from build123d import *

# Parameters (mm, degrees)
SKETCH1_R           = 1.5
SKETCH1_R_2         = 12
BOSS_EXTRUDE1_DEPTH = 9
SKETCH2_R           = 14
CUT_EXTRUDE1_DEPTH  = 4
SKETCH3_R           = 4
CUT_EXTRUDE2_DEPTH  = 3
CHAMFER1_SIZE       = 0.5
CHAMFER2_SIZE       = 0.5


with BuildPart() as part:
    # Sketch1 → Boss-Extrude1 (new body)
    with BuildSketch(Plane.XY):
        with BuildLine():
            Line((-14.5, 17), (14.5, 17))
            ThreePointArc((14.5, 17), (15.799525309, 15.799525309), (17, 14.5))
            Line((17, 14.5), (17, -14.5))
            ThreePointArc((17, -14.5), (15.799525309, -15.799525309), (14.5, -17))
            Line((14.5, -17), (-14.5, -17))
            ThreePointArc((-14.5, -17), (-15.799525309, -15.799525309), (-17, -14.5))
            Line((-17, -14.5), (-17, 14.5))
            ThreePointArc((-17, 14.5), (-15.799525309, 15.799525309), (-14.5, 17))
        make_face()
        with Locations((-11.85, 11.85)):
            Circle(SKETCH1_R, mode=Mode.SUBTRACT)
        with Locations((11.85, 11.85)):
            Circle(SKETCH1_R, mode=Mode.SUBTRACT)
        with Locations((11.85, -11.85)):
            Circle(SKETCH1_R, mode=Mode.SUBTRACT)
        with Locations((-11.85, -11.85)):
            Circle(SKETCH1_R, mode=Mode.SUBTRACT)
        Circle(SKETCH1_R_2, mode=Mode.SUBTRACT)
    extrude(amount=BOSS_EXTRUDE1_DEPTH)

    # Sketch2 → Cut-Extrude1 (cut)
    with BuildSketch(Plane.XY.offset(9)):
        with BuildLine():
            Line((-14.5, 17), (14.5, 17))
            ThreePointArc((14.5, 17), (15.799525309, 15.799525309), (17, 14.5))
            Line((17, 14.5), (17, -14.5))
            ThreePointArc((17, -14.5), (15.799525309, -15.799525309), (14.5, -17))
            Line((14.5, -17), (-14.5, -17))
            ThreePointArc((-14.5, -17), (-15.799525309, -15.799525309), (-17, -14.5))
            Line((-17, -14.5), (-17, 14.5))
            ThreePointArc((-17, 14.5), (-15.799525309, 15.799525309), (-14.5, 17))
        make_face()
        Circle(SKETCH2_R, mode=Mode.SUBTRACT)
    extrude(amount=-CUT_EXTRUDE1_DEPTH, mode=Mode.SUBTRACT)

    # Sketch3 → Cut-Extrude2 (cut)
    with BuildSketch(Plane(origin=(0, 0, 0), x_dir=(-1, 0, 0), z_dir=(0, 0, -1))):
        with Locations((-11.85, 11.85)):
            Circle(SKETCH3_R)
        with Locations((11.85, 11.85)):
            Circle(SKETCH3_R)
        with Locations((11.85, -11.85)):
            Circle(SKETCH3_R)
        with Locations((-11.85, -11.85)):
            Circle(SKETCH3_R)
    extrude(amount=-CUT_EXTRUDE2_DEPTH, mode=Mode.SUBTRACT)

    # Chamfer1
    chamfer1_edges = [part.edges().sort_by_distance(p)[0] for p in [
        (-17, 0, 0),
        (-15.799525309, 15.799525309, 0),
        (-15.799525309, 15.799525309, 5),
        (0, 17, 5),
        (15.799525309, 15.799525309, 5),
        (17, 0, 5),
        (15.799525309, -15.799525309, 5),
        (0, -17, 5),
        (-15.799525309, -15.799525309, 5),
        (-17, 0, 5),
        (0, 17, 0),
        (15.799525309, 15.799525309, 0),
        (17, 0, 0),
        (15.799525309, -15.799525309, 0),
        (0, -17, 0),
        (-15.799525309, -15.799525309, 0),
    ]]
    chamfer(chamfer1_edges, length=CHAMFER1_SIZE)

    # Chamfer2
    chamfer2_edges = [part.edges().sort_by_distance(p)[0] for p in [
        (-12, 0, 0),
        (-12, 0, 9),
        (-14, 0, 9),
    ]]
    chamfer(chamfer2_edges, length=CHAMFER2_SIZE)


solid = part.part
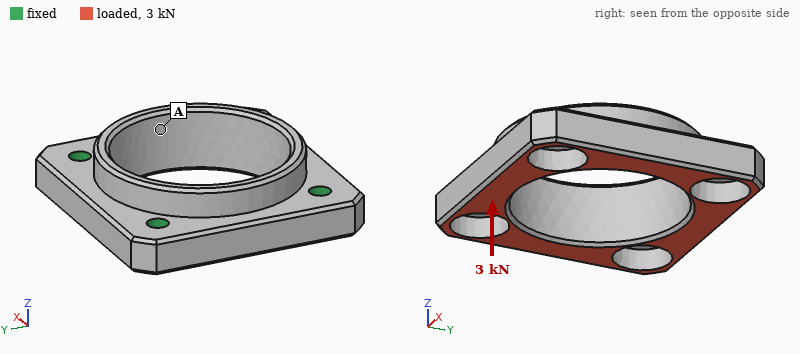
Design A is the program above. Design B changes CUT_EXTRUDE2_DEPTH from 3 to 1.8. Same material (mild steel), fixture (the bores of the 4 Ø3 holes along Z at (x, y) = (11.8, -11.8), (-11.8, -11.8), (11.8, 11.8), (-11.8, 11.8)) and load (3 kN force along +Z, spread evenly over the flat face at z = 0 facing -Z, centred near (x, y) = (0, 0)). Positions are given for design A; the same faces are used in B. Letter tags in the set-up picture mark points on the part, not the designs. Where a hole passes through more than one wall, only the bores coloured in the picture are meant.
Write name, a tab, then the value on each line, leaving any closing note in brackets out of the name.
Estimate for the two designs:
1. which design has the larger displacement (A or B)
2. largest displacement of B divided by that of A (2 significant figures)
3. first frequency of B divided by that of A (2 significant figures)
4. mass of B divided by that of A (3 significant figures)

which design has the larger displacement	A
largest displacement of B divided by that of A	0.75
first frequency of B divided by that of A	1.3
mass of B divided by that of A	1.06
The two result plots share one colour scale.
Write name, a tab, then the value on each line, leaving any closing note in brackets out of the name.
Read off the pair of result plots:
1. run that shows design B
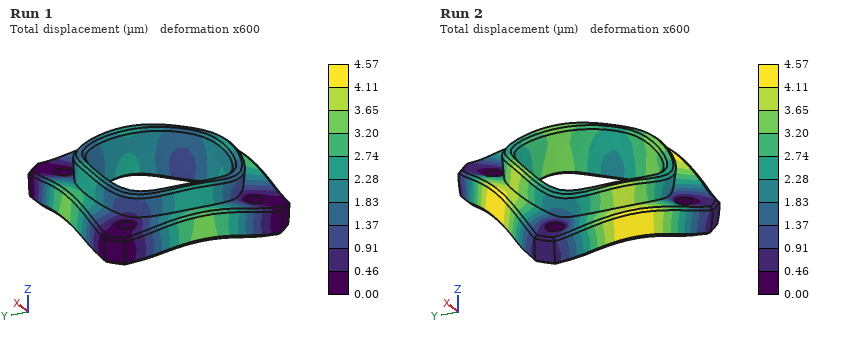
run that shows design B	Run 1
